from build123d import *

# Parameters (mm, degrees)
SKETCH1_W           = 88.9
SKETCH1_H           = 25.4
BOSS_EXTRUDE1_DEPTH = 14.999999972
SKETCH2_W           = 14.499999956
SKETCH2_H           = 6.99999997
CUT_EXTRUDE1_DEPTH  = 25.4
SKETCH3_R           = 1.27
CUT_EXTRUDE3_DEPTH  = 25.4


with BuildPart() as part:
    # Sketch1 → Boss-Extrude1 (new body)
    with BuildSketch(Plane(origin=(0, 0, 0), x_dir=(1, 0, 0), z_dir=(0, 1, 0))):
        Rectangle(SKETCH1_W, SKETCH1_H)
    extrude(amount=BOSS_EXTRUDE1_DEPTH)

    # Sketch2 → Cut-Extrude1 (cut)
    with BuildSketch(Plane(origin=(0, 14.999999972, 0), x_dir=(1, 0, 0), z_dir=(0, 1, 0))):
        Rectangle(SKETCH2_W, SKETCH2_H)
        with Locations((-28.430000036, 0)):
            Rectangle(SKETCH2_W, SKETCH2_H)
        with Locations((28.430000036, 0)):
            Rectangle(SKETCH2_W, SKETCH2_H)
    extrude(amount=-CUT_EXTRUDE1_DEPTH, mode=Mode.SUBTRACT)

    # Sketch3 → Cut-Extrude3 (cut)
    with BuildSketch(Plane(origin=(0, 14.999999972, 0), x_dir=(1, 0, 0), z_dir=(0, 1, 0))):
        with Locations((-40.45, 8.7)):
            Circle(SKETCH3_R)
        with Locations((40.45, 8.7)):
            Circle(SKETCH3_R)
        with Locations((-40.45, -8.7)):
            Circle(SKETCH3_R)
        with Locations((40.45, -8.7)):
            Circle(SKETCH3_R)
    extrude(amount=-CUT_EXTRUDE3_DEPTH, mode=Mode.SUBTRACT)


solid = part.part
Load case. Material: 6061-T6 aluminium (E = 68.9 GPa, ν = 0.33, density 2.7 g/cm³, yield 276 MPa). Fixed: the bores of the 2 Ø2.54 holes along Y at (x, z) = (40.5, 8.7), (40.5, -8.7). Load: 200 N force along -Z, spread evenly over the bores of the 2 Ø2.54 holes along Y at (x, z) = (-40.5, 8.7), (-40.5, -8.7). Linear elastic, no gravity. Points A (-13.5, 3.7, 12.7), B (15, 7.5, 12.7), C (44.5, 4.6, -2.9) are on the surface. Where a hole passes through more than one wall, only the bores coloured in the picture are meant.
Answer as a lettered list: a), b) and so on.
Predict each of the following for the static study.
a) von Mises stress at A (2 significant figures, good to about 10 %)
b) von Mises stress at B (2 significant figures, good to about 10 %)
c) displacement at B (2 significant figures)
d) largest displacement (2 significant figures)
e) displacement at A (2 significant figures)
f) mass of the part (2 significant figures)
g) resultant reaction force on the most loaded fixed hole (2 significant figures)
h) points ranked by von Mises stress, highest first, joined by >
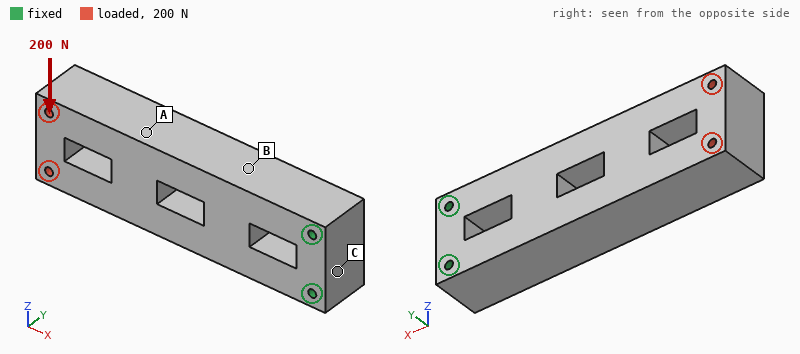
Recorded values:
a) 3.2 MPa
b) 6.7 MPa
c) 6.7 µm
d) 35 µm
e) 19 µm
f) 78 g
g) 870 N
h) B > A > C
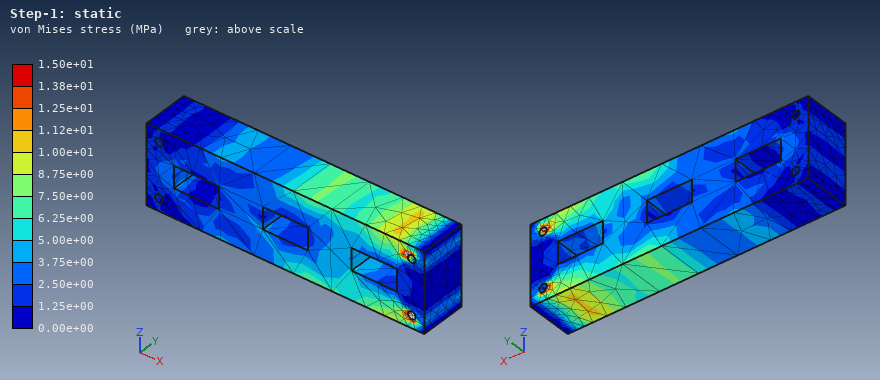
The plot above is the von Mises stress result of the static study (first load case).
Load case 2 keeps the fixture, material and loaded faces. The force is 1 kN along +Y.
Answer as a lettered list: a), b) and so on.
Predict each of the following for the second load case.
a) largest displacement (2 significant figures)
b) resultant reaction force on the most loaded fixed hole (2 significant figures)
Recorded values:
a) 0.53 mm
b) 500 N
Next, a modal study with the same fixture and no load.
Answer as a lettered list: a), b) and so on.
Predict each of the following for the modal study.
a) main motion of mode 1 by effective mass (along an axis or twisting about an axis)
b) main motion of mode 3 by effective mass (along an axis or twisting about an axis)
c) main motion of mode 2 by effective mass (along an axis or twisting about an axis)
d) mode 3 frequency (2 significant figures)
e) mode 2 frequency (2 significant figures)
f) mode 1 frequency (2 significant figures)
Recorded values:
a) along Y
b) twisting about X
c) along Z
d) 6200 Hz
e) 2600 Hz
f) 1500 Hz
